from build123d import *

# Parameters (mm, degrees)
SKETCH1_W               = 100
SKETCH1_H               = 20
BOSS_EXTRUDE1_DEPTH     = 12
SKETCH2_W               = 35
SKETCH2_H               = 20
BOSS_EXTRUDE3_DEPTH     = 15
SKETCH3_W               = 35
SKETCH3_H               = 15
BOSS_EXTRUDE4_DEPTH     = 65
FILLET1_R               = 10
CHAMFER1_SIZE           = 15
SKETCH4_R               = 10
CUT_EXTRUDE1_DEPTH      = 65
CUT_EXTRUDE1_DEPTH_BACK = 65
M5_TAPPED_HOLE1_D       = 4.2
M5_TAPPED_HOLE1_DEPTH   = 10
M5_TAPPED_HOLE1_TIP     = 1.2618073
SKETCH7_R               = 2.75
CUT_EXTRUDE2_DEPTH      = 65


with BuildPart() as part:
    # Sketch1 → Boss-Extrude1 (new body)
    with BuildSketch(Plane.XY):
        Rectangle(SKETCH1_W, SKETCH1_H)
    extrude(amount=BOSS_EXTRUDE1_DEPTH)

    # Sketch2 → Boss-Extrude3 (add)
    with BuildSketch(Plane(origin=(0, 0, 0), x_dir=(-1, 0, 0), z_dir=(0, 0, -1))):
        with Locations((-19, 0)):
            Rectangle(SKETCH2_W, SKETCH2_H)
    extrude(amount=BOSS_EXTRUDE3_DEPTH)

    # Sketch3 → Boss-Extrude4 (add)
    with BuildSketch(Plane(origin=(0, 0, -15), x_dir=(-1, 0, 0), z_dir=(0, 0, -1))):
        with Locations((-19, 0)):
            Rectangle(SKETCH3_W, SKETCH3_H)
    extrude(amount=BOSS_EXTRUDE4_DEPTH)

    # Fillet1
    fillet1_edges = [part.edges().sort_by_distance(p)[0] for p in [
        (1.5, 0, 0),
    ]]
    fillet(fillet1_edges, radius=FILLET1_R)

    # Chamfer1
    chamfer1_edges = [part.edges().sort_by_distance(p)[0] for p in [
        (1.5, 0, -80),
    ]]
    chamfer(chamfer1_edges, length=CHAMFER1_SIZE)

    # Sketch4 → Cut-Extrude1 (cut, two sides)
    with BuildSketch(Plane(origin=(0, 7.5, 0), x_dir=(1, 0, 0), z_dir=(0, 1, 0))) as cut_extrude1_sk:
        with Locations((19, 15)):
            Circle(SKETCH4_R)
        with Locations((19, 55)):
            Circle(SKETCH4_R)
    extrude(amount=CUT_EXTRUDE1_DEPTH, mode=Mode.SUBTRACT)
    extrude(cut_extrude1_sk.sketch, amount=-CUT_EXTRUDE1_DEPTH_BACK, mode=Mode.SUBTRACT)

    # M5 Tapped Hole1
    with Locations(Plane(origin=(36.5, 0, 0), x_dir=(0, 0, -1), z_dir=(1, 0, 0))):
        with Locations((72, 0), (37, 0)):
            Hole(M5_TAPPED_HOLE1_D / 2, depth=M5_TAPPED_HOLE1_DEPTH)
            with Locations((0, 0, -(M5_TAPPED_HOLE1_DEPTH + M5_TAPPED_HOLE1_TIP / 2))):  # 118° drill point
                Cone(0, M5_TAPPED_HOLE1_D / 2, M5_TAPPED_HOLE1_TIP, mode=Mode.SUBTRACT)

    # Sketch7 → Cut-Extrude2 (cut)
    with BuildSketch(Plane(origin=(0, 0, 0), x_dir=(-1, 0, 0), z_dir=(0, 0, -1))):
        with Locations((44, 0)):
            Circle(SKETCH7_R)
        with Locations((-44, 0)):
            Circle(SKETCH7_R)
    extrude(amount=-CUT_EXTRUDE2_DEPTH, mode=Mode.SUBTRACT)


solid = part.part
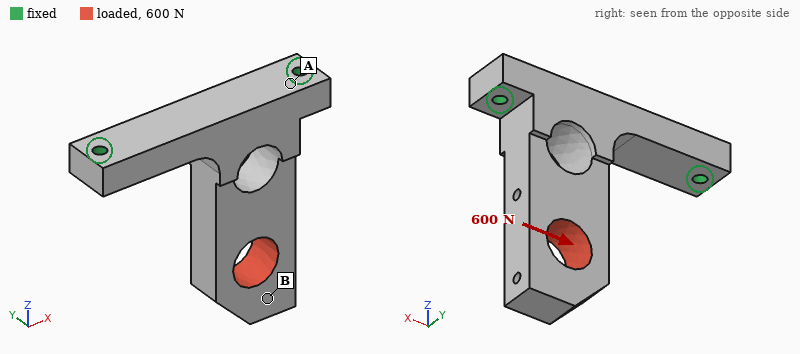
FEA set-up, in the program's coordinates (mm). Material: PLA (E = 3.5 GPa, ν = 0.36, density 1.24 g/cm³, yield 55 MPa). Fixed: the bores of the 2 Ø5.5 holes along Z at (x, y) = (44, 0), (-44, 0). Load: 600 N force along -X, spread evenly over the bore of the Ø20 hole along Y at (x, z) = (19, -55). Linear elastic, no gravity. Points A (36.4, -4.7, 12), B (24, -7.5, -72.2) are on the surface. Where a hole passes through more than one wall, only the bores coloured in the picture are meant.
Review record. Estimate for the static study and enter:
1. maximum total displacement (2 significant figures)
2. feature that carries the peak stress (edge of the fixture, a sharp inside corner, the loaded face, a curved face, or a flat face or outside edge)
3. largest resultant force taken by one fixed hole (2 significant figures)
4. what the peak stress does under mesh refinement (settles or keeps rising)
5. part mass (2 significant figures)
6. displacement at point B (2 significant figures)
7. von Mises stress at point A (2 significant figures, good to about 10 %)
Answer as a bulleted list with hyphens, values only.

- 1.2 mm
- edge of the fixture
- 570 N
- keeps rising
- 70 g
- 1.1 mm
- 11 MPa
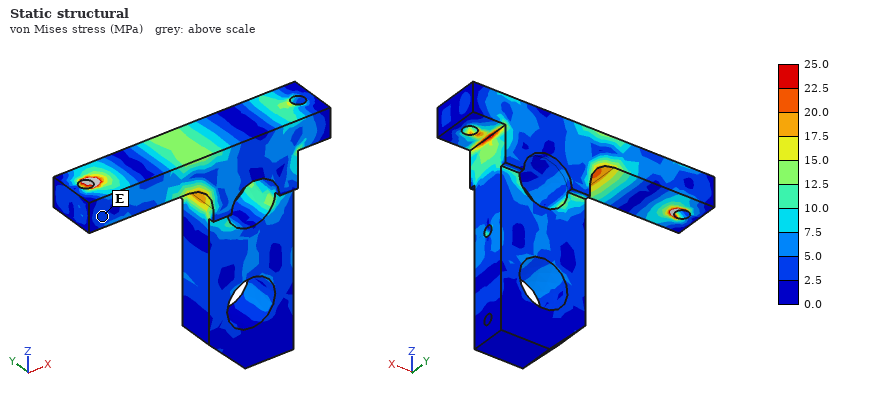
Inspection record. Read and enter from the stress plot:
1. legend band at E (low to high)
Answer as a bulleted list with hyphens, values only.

- 2.5 to 5.0 MPa
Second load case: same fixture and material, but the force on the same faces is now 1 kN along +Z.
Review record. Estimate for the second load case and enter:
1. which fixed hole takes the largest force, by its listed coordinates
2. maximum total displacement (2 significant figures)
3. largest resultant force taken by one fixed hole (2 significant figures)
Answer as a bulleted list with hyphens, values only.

- (44, 0)
- 0.37 mm
- 760 N
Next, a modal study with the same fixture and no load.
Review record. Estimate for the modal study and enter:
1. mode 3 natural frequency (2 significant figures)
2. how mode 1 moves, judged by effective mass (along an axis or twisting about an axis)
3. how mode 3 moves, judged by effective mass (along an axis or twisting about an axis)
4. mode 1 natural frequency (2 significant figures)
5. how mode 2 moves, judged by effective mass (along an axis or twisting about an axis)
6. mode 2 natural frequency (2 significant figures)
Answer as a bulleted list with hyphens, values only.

- 1700 Hz
- along Y
- along Y
- 400 Hz
- along X
- 790 Hz
